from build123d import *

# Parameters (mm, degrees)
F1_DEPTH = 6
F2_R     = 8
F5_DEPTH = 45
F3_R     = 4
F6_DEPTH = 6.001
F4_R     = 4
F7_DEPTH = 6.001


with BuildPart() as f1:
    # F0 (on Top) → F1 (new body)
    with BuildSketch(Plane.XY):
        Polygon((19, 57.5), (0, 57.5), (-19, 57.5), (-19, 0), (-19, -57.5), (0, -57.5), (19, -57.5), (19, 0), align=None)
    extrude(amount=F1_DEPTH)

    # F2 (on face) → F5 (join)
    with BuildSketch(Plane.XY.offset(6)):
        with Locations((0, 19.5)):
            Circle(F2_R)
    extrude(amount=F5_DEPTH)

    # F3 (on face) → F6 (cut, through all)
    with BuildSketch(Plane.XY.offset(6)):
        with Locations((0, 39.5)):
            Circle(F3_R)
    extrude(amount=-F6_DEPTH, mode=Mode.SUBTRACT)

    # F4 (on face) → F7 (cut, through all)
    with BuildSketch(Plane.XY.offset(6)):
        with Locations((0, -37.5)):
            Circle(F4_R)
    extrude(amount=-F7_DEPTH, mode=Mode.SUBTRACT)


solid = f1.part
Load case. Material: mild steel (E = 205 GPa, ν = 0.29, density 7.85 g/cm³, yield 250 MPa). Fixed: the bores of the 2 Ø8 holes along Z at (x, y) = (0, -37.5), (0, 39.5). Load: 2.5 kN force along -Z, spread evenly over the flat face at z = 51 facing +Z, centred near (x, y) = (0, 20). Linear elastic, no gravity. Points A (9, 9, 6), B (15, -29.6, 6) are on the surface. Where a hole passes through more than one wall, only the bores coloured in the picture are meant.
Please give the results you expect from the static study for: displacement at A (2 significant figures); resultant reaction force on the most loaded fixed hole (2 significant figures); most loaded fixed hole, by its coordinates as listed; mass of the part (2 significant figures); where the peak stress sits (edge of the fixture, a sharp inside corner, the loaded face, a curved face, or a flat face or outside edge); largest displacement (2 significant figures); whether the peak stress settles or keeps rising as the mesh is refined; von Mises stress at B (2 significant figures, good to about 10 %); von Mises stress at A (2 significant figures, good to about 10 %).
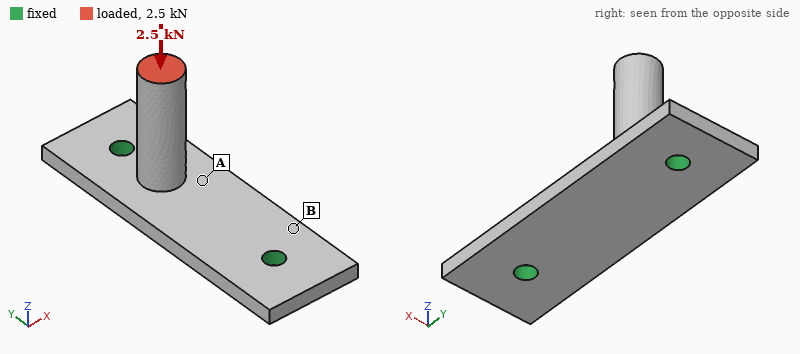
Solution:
23 µm
2.0 kN
(0, 39.5)
270 g
edge of the fixture
50 µm
keeps rising
20 MPa
43 MPa
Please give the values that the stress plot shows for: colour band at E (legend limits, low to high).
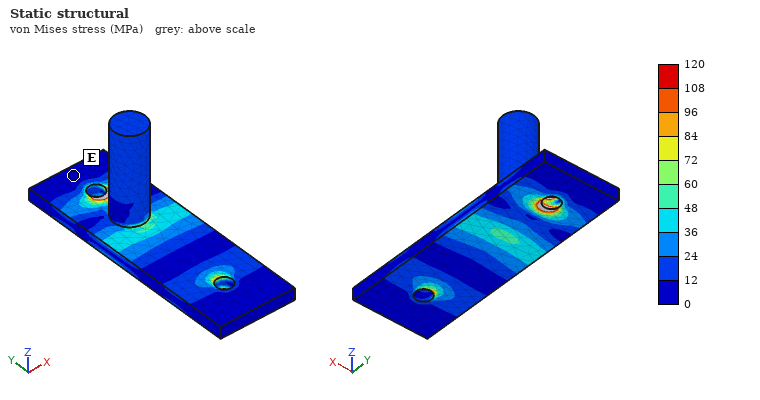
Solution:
0 to 12 MPa
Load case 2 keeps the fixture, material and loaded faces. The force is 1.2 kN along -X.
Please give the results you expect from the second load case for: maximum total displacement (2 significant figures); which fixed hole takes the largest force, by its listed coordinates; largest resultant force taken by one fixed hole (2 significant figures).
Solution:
0.21 mm
(0, 39.5)
940 N
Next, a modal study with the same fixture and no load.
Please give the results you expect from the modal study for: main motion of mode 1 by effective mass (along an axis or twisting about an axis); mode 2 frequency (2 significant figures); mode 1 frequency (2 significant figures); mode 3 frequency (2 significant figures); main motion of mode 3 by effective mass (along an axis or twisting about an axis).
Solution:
along X
2600 Hz
2400 Hz
6200 Hz
along Z
